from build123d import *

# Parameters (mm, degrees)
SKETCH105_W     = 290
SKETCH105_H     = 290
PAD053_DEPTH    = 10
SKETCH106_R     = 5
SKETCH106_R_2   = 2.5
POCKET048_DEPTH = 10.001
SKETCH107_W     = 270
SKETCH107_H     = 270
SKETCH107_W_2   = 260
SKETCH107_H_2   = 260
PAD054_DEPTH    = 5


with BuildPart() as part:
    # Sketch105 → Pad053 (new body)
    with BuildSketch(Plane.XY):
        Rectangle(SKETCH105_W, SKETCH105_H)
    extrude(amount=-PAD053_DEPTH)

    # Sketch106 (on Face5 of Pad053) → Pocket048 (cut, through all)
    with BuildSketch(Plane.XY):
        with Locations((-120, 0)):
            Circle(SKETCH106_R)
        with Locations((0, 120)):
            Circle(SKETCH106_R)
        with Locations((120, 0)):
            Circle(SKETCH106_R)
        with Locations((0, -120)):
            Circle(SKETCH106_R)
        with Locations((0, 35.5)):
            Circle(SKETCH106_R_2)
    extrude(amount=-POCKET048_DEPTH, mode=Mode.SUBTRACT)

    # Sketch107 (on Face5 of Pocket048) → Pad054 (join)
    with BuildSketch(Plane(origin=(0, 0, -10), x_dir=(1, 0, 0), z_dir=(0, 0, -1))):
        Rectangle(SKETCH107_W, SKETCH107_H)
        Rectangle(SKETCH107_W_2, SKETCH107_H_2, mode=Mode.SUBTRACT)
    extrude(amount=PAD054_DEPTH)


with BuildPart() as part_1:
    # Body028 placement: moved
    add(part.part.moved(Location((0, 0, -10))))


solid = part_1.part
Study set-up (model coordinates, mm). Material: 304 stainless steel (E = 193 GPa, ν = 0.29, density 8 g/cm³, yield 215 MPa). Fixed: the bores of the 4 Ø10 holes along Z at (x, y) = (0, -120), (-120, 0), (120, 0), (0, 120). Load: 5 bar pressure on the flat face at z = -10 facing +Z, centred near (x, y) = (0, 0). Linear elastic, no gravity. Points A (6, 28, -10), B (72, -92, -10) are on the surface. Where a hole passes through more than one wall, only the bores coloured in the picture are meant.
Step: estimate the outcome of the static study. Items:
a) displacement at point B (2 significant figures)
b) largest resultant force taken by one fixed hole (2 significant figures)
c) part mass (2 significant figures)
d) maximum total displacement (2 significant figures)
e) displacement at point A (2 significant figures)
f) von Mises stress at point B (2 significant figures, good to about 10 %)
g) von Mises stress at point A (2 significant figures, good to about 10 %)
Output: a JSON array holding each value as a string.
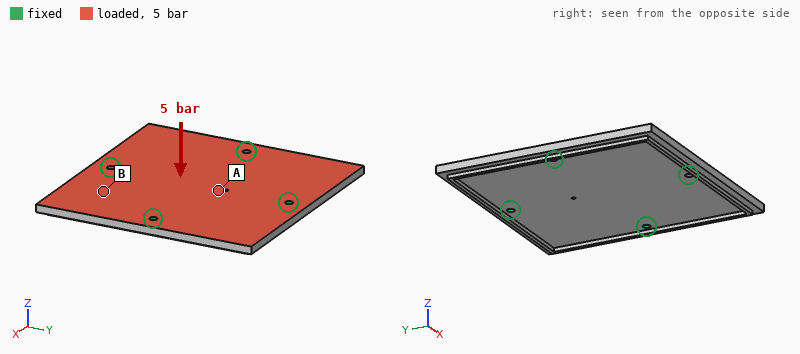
["0.14 mm", "11 kN", "6.9 kg", "0.41 mm", "0.11 mm", "57 MPa", "21 MPa"]
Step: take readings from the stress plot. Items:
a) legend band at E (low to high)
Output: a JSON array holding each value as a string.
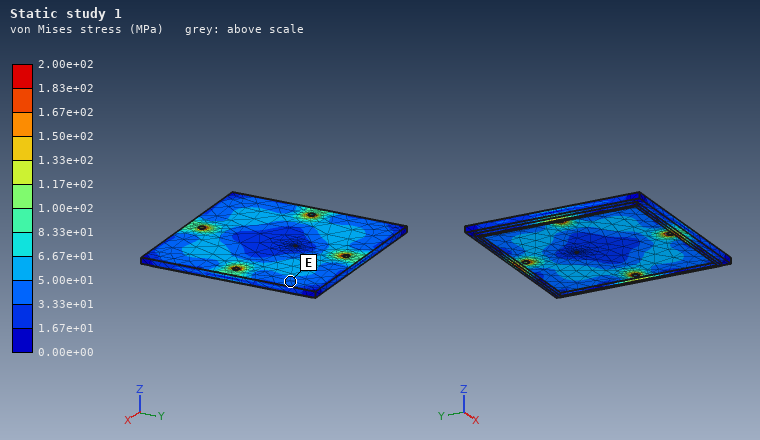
["3.33e+01 to 5.00e+01 MPa"]
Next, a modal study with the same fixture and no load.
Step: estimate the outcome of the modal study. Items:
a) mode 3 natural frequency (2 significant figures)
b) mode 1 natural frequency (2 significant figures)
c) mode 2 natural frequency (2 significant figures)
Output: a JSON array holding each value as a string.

["760 Hz", "700 Hz", "760 Hz"]
